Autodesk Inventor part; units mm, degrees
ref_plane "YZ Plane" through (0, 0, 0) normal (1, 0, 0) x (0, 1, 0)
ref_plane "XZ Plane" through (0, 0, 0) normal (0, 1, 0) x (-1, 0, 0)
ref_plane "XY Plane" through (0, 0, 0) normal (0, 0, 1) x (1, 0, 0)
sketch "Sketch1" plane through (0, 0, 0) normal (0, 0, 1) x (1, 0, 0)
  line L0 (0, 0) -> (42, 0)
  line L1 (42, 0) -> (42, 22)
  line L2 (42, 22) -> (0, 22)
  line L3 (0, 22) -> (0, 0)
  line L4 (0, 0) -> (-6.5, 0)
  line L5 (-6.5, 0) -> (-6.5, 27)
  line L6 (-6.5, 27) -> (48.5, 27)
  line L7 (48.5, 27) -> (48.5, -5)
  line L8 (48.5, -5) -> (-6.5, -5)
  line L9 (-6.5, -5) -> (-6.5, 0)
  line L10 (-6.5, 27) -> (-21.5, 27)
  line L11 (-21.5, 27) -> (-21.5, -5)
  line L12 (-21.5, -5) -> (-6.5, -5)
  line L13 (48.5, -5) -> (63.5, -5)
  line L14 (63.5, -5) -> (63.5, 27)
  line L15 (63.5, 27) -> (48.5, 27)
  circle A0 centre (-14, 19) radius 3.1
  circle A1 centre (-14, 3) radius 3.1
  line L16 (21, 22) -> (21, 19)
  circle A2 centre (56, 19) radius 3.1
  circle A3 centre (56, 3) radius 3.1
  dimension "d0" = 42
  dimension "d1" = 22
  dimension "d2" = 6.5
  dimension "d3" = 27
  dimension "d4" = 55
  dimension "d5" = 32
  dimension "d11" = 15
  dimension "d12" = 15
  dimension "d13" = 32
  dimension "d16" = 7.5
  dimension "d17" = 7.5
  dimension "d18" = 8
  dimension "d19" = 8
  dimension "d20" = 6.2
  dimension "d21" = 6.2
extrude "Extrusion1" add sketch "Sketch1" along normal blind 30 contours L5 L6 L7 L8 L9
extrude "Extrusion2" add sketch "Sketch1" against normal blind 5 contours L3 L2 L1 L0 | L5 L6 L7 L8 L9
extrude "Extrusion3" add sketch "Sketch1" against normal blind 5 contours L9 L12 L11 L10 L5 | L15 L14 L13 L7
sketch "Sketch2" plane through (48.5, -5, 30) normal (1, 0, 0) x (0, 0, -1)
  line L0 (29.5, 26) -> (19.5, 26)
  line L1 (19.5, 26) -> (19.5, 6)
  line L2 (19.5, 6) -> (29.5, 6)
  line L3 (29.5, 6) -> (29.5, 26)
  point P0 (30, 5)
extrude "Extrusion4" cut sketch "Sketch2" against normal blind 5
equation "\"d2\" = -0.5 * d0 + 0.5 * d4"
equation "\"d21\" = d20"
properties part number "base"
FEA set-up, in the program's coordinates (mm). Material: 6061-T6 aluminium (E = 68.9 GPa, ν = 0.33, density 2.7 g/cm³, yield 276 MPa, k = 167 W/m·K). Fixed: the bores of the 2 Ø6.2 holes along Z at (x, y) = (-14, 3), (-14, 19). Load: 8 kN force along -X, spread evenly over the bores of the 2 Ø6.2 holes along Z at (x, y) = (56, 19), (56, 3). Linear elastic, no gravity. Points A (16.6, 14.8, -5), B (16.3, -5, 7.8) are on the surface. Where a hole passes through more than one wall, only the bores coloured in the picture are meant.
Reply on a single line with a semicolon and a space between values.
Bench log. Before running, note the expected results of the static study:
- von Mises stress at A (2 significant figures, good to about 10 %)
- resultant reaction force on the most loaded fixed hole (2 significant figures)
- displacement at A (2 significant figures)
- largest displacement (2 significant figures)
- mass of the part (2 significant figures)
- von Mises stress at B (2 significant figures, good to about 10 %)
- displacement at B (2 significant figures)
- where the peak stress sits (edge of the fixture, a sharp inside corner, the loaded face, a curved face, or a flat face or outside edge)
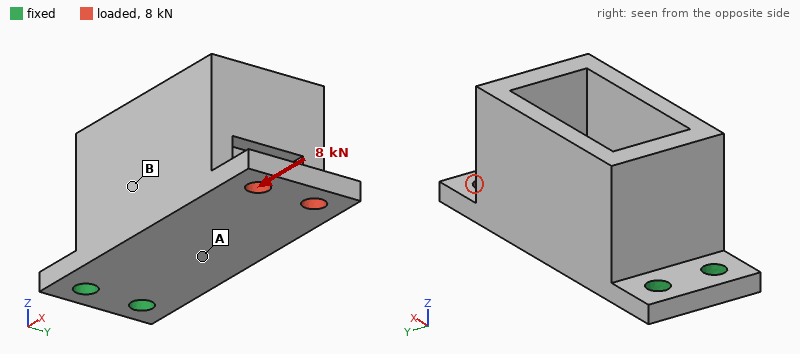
45 MPa; 4.0 kN; 0.028 mm; 0.12 mm; 100 g; 14 MPa; 0.018 mm; the loaded face
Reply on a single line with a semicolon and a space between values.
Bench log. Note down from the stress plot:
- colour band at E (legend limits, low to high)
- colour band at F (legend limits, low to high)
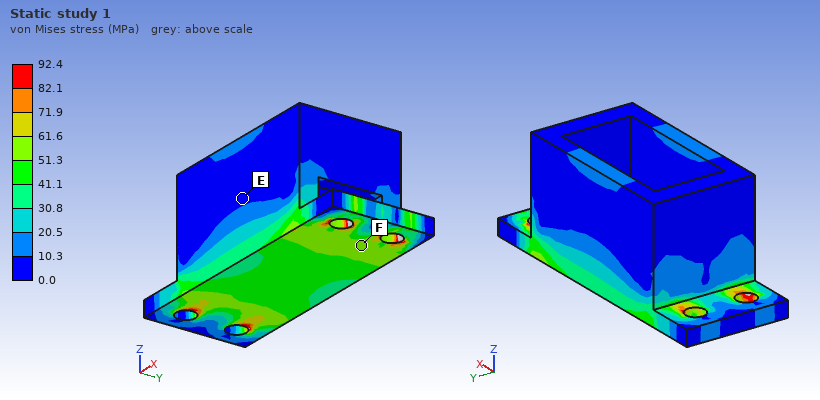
0.0 to 10.3 MPa; 51.3 to 61.6 MPa
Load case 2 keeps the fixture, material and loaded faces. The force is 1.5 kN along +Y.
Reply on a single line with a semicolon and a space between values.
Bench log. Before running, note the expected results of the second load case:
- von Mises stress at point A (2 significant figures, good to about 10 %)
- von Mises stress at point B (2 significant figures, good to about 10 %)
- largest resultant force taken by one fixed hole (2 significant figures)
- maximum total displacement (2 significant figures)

25 MPa; 18 MPa; 5.2 kN; 0.20 mm
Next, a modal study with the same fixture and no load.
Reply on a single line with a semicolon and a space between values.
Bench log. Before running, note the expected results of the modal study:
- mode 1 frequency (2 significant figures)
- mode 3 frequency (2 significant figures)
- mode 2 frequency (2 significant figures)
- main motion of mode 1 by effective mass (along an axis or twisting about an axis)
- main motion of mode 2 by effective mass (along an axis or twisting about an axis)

680 Hz; 3500 Hz; 2300 Hz; along Z; along Y
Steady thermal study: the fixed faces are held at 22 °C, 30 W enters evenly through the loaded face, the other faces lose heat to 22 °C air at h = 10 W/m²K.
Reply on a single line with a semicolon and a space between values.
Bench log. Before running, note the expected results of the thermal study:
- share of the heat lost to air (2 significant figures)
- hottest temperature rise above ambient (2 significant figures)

11 %; 48 K
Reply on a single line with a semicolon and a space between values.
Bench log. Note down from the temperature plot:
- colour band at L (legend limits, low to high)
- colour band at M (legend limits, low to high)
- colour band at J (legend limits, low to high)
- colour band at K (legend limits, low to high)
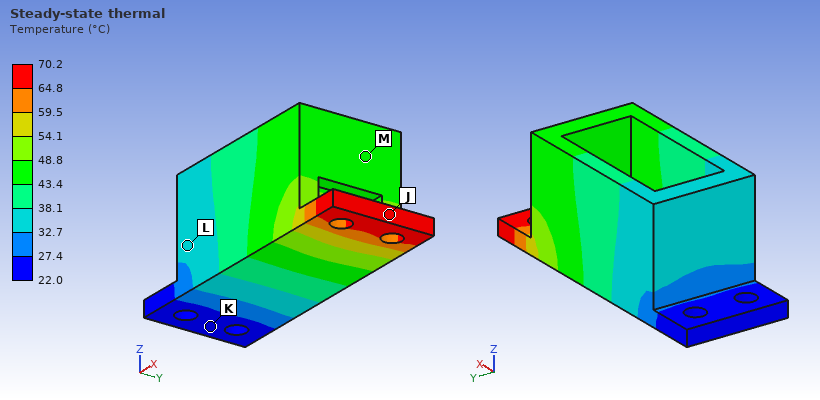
32.7 to 38.1 °C; 43.4 to 48.8 °C; 64.8 to 70.2 °C; 22.0 to 27.4 °C
